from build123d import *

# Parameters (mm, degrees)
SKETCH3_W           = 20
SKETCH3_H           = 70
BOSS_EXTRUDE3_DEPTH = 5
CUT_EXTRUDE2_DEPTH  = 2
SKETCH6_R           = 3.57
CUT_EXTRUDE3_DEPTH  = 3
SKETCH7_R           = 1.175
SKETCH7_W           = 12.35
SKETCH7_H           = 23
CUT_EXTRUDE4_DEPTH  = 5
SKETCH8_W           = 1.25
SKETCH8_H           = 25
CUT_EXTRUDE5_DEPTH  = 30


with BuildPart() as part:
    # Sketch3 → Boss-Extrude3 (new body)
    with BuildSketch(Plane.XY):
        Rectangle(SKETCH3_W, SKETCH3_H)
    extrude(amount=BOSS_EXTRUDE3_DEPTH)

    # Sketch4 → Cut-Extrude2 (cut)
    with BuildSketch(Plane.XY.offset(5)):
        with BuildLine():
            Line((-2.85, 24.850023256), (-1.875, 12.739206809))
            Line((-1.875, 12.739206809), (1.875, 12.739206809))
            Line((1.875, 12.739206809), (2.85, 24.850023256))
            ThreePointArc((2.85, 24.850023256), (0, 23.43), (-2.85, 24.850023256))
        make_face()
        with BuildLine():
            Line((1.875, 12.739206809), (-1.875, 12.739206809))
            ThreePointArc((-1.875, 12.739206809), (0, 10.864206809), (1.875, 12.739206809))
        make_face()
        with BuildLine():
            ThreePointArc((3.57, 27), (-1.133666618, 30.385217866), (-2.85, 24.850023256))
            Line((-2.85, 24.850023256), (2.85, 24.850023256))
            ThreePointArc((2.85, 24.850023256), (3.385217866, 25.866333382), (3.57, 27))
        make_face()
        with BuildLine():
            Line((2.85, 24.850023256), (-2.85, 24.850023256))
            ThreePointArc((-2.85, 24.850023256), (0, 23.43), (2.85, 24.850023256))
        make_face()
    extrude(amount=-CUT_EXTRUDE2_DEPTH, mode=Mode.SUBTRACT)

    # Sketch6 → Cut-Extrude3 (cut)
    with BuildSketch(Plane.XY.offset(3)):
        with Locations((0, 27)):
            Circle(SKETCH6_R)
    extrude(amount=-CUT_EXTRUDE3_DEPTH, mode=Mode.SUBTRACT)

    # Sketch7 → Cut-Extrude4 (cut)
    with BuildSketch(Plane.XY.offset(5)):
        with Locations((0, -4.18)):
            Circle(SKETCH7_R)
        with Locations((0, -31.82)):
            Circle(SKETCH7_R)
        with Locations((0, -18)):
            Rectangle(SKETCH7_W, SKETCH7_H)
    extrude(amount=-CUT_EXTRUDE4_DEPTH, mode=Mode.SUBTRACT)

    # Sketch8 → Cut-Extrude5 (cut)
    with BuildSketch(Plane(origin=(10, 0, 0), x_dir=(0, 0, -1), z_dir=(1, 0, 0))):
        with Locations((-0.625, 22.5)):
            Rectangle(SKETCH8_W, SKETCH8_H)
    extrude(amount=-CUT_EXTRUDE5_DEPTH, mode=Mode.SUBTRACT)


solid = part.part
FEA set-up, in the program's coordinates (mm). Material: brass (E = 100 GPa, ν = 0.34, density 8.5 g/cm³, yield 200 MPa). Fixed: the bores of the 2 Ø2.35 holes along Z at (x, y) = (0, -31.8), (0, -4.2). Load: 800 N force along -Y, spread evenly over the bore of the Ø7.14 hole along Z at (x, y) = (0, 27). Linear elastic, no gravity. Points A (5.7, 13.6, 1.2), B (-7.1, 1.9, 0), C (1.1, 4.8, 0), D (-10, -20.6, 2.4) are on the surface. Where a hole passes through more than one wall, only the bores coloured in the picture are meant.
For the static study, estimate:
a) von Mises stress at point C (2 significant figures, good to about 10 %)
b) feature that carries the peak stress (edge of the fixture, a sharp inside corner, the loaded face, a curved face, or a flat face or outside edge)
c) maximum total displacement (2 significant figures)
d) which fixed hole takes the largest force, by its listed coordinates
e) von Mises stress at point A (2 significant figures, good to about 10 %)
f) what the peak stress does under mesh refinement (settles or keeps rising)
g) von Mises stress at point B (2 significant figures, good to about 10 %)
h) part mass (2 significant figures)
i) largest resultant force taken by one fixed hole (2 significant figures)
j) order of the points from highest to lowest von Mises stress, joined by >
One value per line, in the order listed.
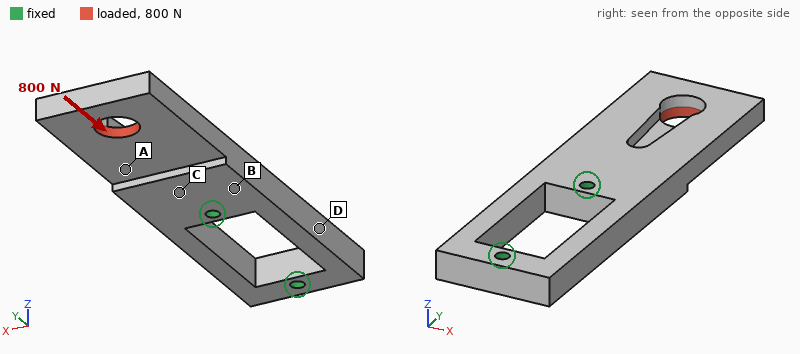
14 MPa
edge of the fixture
38 µm
(0, -4.2)
27 MPa
keeps rising
9.5 MPa
39 g
730 N
A > C > B > D
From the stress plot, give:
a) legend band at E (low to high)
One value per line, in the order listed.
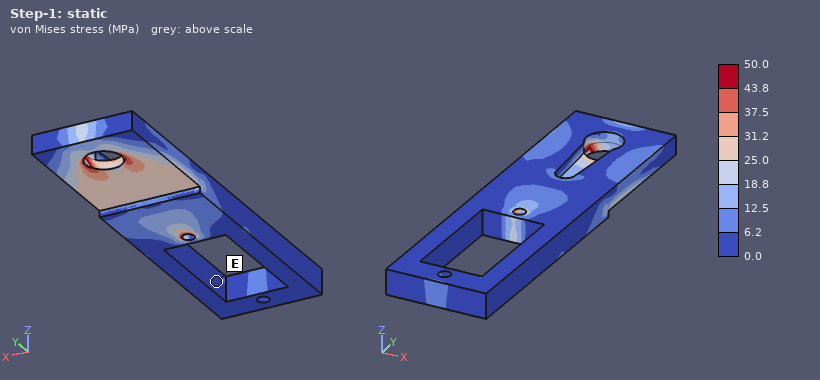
0.0 to 6.2 MPa
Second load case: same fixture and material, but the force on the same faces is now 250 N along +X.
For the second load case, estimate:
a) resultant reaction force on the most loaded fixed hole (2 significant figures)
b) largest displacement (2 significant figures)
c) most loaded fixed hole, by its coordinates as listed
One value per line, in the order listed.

330 N
63 µm
(0, -4.2)
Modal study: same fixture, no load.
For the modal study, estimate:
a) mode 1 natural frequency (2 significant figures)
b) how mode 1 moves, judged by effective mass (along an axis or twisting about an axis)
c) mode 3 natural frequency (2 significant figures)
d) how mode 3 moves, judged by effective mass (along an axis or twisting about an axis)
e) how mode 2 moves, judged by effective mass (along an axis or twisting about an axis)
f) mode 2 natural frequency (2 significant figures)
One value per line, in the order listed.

1800 Hz
along Z
5100 Hz
twisting about Y
along X
3300 Hz
